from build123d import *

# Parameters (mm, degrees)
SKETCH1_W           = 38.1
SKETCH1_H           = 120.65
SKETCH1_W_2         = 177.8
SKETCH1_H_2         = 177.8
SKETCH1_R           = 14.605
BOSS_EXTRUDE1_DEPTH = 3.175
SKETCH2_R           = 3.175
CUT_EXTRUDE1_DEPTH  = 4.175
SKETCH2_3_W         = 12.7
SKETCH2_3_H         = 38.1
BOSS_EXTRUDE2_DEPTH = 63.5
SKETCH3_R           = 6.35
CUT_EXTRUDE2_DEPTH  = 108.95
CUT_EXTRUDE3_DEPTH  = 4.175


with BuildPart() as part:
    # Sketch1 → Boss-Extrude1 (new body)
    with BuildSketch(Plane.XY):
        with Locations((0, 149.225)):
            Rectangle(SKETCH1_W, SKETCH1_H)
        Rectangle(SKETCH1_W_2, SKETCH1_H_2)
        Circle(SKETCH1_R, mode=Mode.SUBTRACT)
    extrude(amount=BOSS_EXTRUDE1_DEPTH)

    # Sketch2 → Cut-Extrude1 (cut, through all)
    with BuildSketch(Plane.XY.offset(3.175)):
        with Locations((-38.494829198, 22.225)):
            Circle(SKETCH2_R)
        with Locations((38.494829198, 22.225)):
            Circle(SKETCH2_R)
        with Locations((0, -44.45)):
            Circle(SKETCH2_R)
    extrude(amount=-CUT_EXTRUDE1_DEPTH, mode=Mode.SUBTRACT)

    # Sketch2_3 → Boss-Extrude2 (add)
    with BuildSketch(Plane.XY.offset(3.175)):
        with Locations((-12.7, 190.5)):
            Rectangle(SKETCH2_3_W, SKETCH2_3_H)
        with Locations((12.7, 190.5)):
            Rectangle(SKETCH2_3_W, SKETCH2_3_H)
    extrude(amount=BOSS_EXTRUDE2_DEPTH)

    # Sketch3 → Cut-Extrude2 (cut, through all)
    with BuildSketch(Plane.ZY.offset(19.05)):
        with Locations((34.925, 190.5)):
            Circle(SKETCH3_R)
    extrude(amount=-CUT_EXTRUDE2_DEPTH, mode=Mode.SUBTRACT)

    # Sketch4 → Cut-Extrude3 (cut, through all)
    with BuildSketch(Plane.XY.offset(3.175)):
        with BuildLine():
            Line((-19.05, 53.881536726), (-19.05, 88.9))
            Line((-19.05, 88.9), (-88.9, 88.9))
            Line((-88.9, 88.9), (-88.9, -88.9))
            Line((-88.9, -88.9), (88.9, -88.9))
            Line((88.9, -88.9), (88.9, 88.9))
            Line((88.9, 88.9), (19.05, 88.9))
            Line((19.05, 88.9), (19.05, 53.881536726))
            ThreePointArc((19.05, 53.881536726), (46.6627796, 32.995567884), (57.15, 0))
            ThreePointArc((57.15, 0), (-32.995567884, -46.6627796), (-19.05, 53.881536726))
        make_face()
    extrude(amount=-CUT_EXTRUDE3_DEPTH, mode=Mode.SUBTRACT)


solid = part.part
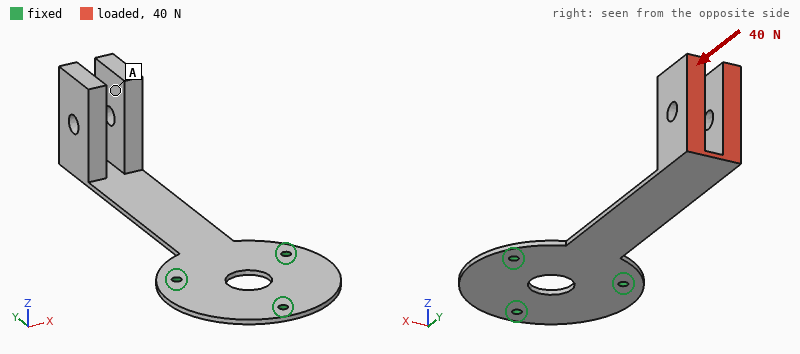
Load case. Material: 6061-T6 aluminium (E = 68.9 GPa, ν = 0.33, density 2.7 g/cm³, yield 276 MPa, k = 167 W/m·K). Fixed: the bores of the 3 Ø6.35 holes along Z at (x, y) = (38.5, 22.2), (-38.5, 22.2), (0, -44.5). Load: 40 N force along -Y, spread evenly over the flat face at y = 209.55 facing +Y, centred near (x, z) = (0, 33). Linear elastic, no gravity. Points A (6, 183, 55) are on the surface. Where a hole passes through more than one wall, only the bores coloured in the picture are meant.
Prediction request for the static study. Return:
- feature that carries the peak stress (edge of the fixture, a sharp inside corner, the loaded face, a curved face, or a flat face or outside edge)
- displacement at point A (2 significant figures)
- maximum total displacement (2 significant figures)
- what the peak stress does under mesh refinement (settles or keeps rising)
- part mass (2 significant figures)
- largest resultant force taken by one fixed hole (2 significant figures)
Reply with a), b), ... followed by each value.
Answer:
a) a sharp inside corner
b) 2.4 mm
c) 3.1 mm
d) keeps rising
e) 290 g
f) 20 N
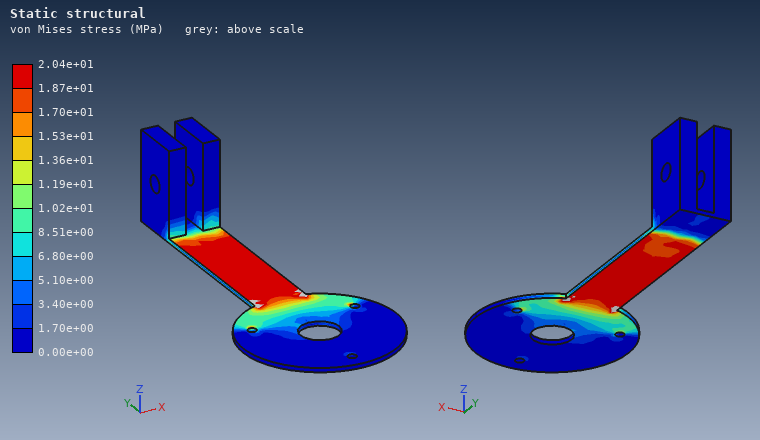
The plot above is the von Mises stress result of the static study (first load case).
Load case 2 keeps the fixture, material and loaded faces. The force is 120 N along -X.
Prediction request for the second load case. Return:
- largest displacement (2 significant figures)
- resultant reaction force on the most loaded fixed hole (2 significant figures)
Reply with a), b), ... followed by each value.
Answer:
a) 3.2 mm
b) 300 N
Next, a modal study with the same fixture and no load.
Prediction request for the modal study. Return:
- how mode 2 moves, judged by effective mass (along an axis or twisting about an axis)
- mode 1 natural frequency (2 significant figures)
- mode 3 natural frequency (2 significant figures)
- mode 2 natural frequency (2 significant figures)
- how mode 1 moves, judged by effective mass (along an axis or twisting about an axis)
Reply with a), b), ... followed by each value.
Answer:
a) along X
b) 26 Hz
c) 160 Hz
d) 88 Hz
e) along Z
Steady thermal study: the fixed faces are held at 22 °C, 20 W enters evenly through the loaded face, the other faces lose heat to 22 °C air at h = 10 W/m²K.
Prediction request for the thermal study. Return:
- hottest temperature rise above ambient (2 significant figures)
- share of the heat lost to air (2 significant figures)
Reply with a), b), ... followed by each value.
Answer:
a) 66 K
b) 65 %
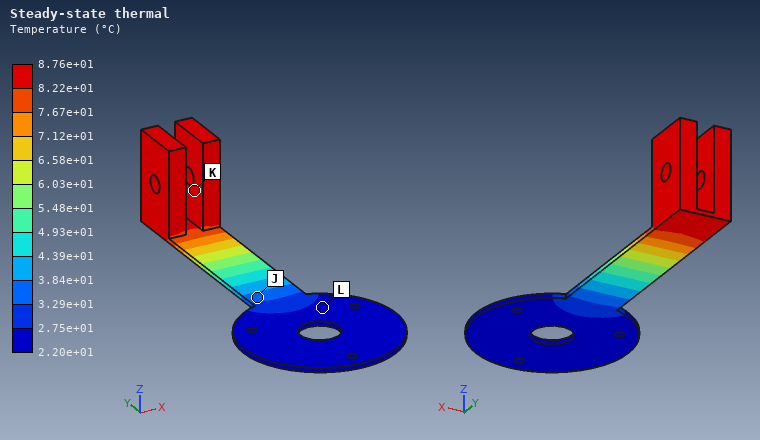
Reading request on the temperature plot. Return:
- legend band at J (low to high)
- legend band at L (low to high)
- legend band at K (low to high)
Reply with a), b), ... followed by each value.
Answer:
a) 3.29e+01 to 3.84e+01 °C
b) 2.20e+01 to 2.75e+01 °C
c) 8.22e+01 to 8.76e+01 °C
